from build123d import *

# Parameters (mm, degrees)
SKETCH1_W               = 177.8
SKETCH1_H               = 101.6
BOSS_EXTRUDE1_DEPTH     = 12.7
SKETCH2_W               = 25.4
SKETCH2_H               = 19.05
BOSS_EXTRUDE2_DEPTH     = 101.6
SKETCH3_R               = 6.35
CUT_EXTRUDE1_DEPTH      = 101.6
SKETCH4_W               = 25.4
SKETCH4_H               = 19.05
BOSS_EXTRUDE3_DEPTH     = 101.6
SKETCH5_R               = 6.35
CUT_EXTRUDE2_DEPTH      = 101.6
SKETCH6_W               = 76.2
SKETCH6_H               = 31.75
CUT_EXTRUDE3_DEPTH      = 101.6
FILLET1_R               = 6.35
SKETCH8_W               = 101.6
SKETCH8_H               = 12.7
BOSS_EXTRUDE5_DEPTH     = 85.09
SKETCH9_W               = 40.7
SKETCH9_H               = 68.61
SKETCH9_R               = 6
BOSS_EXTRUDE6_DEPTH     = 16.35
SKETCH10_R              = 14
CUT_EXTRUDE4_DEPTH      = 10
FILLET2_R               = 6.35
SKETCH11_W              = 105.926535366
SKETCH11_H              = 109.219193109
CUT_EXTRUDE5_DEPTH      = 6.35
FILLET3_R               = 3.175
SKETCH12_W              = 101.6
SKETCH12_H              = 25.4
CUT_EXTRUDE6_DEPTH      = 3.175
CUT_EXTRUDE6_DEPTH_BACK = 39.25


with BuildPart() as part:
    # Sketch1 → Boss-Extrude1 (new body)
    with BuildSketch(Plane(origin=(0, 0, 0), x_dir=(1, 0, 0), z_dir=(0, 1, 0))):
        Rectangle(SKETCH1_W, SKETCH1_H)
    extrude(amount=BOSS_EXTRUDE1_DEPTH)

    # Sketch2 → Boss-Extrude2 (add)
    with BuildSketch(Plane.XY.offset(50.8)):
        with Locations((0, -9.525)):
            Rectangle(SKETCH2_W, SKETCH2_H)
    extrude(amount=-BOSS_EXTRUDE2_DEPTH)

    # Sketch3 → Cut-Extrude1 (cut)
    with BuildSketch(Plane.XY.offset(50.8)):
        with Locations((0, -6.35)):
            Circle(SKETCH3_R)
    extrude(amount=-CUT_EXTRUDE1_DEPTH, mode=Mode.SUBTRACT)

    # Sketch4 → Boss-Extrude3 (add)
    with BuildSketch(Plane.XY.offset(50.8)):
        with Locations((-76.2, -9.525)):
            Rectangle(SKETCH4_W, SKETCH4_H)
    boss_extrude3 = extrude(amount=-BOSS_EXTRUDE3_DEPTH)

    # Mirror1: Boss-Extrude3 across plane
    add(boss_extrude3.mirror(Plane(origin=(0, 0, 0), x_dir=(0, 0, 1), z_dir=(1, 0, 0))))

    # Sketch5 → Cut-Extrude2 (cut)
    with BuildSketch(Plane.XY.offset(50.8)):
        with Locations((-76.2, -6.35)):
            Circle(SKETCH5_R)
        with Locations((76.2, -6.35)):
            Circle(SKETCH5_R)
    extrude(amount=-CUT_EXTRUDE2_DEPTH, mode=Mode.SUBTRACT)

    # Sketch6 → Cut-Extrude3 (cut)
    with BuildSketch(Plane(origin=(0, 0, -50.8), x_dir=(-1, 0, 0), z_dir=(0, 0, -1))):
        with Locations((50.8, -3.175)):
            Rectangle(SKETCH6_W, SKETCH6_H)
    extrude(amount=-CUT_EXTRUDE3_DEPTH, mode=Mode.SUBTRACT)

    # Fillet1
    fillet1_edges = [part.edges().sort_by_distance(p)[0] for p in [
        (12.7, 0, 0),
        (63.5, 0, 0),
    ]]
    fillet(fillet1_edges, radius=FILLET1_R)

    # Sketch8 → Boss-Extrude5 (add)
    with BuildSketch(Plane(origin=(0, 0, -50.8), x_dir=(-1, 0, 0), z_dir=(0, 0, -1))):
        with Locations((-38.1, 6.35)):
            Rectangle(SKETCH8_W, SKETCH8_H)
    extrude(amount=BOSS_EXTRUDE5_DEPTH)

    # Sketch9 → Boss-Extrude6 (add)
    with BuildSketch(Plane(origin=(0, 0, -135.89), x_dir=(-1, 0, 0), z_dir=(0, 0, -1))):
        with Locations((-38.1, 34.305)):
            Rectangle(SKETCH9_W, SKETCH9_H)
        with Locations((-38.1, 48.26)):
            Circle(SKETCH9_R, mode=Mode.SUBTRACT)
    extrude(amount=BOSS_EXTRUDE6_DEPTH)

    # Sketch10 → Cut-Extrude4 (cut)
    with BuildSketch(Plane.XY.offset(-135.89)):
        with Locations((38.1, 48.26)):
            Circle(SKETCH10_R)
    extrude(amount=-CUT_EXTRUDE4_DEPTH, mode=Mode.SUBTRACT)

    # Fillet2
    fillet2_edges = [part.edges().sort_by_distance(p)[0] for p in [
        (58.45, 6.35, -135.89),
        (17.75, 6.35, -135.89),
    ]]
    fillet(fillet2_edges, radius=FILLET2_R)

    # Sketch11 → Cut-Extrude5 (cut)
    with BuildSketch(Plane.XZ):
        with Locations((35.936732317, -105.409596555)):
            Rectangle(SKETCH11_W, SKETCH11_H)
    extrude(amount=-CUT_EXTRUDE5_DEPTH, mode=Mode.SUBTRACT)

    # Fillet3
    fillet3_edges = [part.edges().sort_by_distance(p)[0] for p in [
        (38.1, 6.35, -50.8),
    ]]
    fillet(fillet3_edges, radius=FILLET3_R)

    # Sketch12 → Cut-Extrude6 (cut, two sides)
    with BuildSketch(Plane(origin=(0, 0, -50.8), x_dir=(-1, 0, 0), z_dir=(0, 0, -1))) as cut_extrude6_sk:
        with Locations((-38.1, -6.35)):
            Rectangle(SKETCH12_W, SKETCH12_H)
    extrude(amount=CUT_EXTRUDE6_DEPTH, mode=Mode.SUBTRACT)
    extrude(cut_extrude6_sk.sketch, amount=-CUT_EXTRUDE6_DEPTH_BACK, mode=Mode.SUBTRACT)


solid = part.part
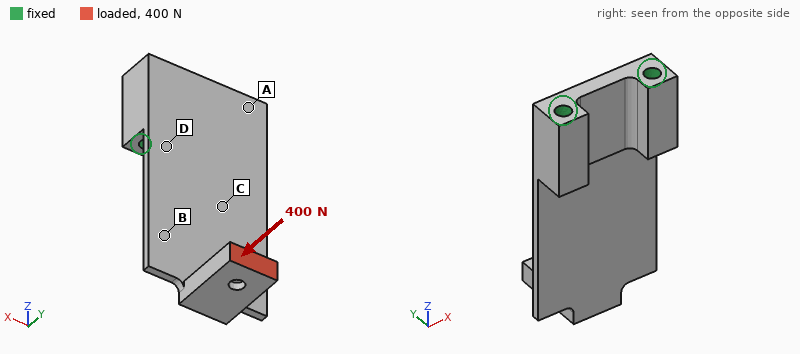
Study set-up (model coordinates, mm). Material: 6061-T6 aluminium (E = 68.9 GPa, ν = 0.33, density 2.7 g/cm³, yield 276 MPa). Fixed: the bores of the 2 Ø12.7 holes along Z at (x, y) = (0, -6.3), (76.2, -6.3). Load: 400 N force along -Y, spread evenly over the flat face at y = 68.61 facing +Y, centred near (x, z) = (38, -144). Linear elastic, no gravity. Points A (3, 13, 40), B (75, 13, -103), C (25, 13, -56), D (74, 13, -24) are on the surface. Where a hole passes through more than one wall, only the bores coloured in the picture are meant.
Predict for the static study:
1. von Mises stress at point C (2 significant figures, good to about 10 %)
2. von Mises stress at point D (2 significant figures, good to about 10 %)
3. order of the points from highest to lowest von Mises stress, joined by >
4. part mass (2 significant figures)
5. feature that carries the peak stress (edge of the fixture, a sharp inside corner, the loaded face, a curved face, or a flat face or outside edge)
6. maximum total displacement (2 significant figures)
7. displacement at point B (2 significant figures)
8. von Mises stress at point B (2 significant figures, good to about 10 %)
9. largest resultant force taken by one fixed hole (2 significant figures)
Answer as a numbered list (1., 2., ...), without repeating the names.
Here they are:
1. 47 MPa
2. 64 MPa
3. D > C > B > A
4. 650 g
5. a flat face or outside edge
6. 2.8 mm
7. 1.2 mm
8. 24 MPa
9. 350 N
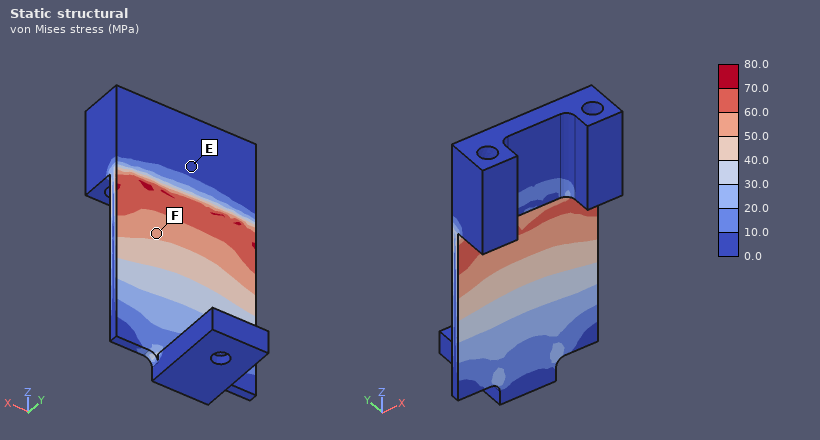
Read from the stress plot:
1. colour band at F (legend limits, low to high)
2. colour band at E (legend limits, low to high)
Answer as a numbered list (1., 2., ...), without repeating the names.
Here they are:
1. 50.0 to 60.0 MPa
2. 0.0 to 10.0 MPa
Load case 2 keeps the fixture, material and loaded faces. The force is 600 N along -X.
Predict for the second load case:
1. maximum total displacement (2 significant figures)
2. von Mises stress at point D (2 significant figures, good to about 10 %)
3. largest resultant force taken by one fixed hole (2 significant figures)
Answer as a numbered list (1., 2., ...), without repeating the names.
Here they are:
1. 1.2 mm
2. 31 MPa
3. 1.2 kN
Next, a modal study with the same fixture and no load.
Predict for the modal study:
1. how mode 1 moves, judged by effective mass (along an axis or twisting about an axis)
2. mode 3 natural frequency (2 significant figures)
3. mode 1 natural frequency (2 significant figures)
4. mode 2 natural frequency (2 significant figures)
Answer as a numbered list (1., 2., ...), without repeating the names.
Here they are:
1. along Y
2. 810 Hz
3. 180 Hz
4. 560 Hz
